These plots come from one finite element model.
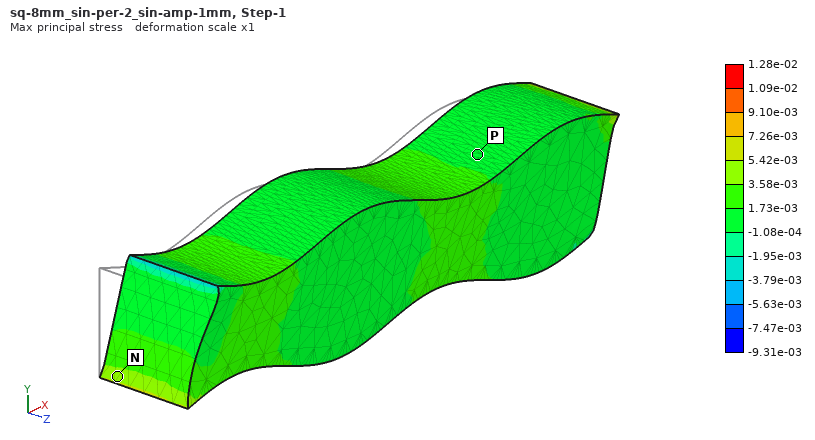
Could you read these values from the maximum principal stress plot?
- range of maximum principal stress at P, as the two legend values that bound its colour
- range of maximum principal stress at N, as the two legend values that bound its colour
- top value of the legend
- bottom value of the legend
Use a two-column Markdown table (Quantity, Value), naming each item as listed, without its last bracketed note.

| Quantity | Value |
|---|---|
| range of maximum principal stress at P, as the two legend values that bound its colour | -1.08e-04 to 1.73e-03 |
| range of maximum principal stress at N, as the two legend values that bound its colour | 3.58e-03 to 5.42e-03 |
| top value of the legend | 1.28e-02 |
| bottom value of the legend | -9.31e-03 |
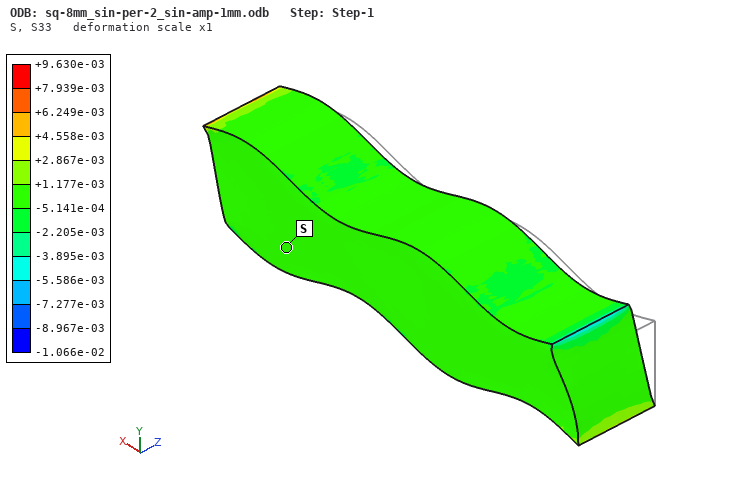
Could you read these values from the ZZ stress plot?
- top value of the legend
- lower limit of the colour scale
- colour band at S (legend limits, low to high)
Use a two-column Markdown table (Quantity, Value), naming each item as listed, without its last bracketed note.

| Quantity | Value |
|---|---|
| top value of the legend | +9.630e-03 |
| lower limit of the colour scale | -1.066e-02 |
| colour band at S | -5.141e-04 to +1.177e-03 |
